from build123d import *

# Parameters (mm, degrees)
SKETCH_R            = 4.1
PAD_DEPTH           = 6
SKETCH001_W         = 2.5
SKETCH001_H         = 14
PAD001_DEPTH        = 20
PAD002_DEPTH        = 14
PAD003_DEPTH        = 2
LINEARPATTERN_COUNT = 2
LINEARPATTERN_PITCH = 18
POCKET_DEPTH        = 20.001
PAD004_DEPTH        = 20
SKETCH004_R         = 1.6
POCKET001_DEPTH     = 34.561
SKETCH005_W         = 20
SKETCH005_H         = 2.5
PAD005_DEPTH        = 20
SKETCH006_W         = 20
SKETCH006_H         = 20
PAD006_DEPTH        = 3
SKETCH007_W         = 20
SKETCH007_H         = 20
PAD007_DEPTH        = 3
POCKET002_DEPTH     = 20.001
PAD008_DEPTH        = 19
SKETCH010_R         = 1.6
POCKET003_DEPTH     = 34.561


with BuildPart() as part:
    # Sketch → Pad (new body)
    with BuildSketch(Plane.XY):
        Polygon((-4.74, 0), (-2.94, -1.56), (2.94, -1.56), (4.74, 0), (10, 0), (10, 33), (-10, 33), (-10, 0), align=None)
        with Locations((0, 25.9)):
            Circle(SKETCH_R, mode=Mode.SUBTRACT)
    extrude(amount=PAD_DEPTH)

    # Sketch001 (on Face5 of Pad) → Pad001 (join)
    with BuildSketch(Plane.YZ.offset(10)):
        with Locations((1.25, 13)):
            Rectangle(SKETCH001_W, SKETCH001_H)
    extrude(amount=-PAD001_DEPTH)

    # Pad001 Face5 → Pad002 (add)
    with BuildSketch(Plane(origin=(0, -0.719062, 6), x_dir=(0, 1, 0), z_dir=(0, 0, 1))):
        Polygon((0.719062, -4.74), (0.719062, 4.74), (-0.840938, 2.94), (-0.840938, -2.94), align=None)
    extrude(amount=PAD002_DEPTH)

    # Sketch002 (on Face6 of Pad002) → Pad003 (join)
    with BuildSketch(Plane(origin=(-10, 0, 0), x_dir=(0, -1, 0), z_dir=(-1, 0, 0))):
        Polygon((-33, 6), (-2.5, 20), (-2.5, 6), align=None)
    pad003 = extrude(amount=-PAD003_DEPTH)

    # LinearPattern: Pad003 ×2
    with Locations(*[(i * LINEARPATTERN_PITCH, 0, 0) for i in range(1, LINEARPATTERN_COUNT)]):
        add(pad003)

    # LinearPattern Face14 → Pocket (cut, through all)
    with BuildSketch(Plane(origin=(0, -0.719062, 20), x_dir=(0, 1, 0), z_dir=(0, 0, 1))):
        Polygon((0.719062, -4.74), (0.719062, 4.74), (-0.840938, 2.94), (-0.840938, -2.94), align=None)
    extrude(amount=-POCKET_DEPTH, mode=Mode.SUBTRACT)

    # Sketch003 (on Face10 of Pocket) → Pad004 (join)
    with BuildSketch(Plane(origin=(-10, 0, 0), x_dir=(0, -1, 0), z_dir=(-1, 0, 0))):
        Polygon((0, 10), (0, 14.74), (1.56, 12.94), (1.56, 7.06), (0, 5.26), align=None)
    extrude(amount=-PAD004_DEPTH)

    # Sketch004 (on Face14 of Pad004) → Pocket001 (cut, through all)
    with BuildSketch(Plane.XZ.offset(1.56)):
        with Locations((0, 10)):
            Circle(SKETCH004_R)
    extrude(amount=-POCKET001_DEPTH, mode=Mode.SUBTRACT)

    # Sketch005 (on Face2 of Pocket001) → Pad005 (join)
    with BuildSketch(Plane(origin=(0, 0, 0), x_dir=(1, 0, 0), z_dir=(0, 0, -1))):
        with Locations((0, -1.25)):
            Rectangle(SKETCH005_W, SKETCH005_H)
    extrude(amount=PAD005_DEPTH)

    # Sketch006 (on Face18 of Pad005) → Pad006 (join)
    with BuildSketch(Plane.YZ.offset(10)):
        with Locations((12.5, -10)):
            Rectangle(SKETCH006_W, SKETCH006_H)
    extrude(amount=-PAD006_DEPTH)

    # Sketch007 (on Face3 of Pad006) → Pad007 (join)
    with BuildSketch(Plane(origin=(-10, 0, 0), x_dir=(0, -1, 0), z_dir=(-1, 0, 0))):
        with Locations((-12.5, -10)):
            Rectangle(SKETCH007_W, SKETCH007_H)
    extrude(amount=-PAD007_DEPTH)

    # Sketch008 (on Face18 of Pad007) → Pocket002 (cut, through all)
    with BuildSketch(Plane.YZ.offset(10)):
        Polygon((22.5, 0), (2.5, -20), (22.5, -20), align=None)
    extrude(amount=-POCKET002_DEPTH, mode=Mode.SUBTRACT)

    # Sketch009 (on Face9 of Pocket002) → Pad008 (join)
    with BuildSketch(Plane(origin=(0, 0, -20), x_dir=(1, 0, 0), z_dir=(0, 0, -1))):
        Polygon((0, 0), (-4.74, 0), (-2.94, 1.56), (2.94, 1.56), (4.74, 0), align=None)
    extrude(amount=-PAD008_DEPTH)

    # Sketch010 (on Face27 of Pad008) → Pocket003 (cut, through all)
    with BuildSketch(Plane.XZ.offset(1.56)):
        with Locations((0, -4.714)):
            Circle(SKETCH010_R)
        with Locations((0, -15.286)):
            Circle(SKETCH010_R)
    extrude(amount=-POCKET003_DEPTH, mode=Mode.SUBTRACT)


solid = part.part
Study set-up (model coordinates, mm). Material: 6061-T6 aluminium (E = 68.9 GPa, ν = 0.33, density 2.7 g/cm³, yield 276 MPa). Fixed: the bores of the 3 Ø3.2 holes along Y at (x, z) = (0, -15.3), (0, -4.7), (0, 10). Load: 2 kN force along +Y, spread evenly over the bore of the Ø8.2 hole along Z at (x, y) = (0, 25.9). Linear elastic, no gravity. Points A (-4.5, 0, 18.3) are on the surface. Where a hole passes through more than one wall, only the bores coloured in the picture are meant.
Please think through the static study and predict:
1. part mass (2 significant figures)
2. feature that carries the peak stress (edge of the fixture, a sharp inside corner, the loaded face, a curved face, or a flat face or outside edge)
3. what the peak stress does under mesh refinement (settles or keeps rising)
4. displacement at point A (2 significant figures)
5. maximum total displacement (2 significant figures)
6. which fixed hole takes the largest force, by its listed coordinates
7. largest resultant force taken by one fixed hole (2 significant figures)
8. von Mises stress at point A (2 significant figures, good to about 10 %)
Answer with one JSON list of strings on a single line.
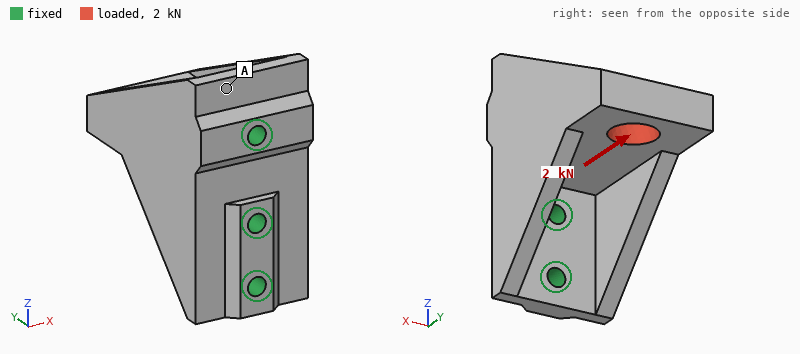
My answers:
["21 g", "edge of the fixture", "keeps rising", "3.8 µm", "17 µm", "(0, 10)", "1.2 kN", "13 MPa"]
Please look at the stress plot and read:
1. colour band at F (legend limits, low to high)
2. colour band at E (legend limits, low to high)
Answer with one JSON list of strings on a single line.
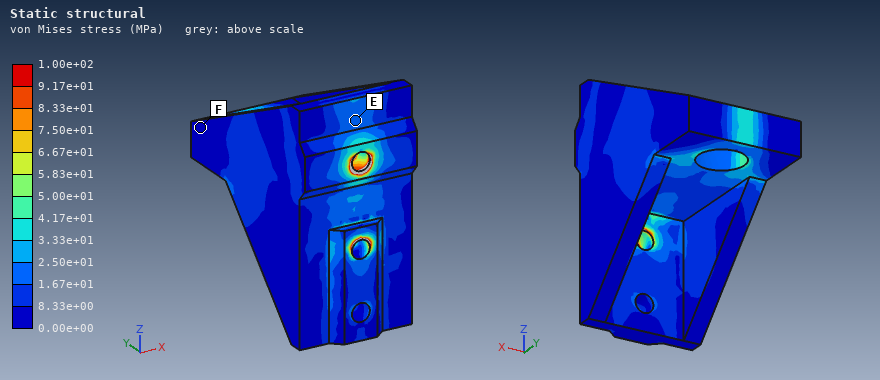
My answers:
["0.00e+00 to 8.33e+00 MPa", "1.67e+01 to 2.50e+01 MPa"]
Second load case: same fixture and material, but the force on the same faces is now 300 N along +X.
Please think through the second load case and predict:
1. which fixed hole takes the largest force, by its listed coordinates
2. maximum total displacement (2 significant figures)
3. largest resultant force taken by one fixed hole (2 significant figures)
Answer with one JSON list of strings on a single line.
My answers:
["(0, -4.7)", "55 µm", "260 N"]
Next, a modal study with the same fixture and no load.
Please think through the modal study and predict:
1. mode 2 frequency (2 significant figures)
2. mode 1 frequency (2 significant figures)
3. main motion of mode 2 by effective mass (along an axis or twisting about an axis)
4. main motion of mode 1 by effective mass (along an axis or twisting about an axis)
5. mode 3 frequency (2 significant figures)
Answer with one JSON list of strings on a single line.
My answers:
["9200 Hz", "5100 Hz", "along Z", "along X", "15 kHz"]
